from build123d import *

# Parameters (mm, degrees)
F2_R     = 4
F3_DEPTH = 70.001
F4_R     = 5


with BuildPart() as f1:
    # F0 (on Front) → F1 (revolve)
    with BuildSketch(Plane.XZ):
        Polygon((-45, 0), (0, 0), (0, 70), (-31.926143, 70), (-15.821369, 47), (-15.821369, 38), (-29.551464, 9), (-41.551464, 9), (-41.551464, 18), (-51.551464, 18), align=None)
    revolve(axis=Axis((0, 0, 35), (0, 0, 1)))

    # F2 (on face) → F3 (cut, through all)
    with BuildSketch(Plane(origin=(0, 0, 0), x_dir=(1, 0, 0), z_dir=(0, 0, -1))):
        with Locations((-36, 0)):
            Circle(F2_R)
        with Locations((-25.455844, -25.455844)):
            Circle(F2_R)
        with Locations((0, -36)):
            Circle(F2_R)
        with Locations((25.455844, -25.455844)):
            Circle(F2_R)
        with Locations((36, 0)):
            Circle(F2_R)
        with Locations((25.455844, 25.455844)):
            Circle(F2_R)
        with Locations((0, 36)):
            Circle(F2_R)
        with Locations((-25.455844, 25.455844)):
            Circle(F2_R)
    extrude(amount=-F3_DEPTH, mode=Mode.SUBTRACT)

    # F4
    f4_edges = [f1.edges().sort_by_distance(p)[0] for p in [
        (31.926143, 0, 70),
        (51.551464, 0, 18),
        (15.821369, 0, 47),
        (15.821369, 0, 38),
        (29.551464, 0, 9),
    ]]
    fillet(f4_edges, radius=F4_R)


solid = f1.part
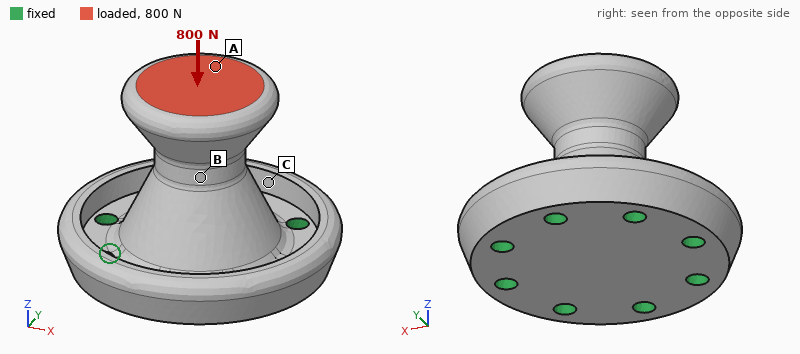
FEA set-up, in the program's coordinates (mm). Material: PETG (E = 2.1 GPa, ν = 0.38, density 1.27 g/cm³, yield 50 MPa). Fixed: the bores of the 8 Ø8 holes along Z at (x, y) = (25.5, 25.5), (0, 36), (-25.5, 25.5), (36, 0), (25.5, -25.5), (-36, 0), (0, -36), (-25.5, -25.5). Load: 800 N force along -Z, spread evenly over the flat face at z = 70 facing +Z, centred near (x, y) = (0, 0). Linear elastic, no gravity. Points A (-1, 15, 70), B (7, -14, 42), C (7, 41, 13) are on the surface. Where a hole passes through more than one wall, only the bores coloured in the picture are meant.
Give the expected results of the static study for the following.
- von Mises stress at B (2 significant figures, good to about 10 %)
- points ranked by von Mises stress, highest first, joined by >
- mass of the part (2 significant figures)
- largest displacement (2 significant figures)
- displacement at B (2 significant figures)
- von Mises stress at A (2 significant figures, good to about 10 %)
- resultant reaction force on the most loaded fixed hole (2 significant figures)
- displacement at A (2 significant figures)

1.2 MPa
B > A > C
220 g
30 µm
20 µm
0.48 MPa
120 N
30 µm
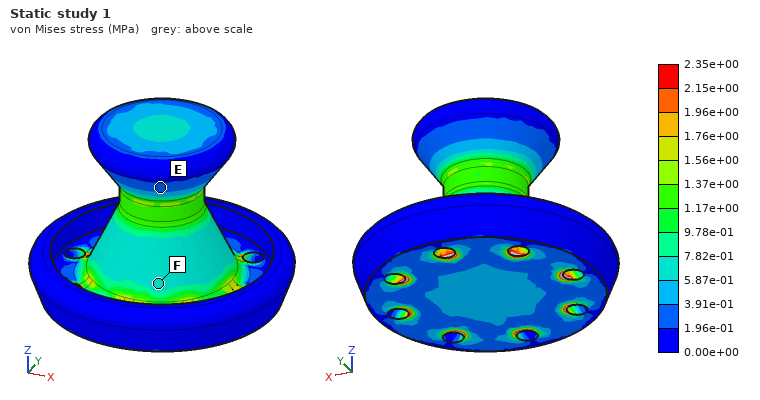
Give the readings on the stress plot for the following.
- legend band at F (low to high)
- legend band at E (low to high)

5.87e-01 to 7.82e-01 MPa
1.96e-01 to 3.91e-01 MPa
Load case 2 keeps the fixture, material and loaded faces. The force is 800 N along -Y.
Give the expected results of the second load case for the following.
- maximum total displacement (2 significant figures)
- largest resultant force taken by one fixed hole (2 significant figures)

0.38 mm
470 N
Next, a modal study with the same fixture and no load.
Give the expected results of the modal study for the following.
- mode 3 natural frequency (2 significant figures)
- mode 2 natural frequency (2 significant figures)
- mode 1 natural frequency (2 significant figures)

2200 Hz
1300 Hz
1300 Hz
